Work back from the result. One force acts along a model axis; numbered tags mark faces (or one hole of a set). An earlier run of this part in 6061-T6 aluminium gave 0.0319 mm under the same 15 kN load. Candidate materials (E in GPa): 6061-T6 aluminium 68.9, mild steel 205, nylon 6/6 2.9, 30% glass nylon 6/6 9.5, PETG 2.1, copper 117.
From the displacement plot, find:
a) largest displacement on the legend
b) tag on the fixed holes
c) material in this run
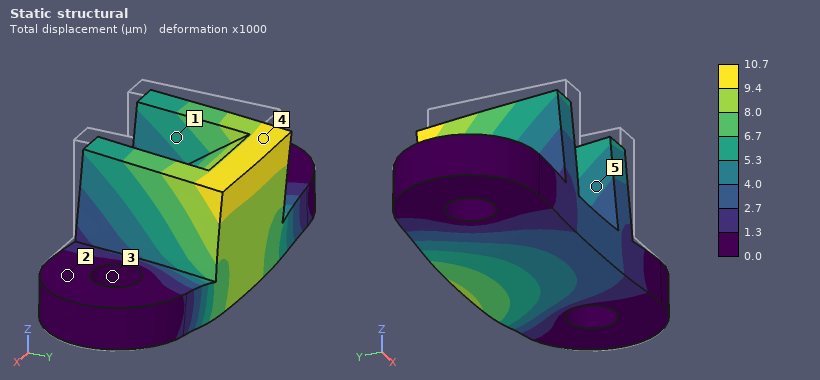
10.7 µm
3
mild steel
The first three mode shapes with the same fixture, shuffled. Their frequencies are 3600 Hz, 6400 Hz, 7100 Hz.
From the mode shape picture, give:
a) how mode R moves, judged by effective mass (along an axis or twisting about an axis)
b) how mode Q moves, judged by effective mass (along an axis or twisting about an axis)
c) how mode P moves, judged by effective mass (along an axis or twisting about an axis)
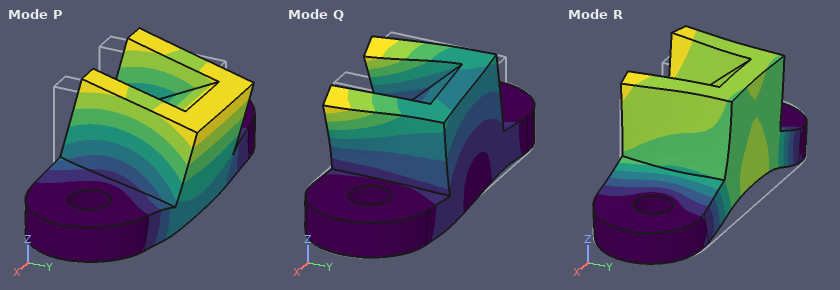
along Z
along X
along Y
